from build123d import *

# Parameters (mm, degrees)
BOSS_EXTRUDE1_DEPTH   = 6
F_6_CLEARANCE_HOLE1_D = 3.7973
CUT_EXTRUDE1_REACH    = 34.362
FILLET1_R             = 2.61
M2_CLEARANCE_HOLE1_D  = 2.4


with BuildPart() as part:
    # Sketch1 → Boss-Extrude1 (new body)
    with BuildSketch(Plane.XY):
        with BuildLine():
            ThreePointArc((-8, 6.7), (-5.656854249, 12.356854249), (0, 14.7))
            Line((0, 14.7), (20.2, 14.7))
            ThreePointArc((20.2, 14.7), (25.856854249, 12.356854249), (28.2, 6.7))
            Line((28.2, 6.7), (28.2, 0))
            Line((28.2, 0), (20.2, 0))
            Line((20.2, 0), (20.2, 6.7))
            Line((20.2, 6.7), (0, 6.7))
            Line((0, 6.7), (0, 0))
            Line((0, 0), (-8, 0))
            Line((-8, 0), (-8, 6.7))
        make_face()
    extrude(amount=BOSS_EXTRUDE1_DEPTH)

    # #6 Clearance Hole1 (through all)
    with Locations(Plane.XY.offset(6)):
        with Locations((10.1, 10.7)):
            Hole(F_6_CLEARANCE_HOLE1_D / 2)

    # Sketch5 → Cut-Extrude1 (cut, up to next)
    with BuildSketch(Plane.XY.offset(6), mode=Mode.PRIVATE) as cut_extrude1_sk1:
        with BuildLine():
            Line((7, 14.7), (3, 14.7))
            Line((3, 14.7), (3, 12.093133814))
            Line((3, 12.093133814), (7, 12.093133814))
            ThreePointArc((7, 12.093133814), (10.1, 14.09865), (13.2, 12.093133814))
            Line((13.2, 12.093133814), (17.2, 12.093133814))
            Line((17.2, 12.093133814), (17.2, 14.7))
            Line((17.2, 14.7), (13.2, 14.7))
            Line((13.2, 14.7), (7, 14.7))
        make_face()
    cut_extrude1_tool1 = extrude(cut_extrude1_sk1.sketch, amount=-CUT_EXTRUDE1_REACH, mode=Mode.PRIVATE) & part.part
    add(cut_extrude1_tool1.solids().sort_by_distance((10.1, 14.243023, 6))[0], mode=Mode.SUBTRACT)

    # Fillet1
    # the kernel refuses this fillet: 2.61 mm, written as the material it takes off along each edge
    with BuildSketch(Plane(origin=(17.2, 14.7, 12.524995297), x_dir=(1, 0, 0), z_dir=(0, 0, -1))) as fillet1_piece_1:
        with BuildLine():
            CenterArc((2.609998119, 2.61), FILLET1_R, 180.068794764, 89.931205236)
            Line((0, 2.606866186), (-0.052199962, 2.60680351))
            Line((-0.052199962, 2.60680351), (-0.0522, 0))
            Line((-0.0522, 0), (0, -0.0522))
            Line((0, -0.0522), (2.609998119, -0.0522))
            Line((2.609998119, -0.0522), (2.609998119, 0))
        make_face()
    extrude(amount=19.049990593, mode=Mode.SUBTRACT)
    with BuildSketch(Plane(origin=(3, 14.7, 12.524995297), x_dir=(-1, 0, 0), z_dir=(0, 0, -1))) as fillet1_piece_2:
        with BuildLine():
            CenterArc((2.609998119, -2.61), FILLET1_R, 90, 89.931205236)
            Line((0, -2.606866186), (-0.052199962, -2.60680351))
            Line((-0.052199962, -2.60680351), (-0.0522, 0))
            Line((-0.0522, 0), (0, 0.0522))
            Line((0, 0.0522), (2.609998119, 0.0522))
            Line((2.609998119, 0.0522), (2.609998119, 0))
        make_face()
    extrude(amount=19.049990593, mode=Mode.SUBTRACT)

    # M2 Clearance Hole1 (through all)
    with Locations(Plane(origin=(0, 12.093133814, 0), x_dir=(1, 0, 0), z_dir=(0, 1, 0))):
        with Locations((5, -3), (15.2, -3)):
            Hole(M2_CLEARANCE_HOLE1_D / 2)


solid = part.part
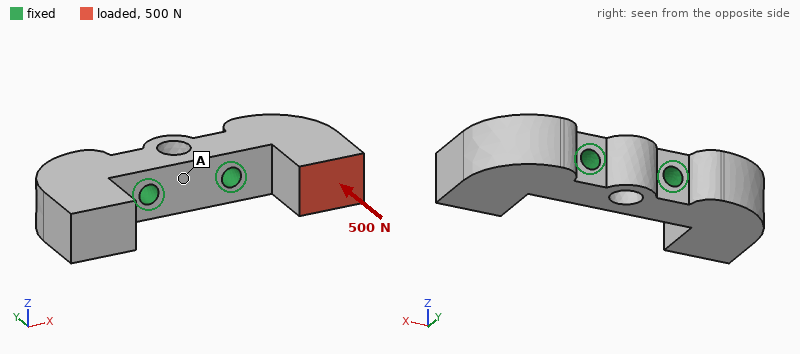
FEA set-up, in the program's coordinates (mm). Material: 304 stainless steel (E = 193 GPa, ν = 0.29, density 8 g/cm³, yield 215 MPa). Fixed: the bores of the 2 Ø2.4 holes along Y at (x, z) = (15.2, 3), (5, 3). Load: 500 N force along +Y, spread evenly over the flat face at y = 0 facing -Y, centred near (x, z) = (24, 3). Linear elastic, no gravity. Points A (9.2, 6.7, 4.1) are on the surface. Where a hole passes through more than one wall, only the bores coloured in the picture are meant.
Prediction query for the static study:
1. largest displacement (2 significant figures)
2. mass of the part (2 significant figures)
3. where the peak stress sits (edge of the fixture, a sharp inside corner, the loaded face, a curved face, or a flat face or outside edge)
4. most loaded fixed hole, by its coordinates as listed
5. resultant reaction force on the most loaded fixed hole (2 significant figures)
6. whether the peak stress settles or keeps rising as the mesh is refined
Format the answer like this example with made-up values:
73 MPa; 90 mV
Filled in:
16 µm; 15 g; edge of the fixture; (15.2, 3); 520 N; keeps rising
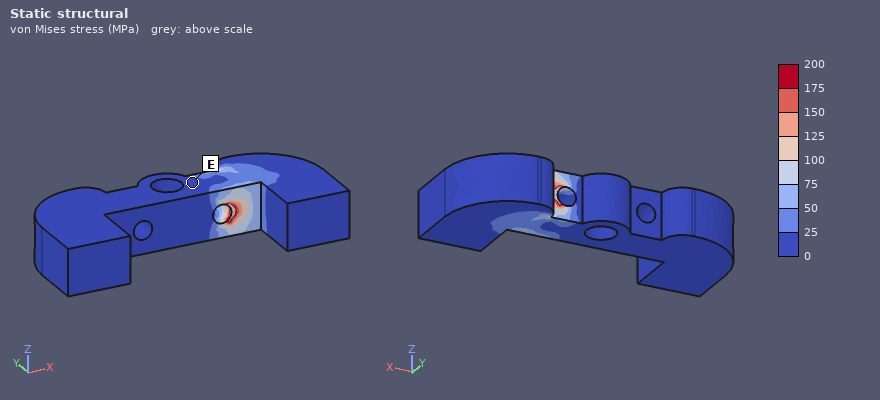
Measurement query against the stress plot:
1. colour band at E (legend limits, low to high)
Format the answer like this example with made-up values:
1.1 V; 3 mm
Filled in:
0 to 25 MPa
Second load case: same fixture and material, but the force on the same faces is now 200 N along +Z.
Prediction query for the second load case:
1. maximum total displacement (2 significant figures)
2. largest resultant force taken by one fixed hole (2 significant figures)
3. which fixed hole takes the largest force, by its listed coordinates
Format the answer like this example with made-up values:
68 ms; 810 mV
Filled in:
16 µm; 250 N; (15.2, 3)
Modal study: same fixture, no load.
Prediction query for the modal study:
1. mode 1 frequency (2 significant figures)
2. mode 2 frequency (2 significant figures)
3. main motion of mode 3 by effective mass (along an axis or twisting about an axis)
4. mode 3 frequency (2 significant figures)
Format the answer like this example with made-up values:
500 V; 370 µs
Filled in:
13 kHz; 14 kHz; along Y; 15 kHz
